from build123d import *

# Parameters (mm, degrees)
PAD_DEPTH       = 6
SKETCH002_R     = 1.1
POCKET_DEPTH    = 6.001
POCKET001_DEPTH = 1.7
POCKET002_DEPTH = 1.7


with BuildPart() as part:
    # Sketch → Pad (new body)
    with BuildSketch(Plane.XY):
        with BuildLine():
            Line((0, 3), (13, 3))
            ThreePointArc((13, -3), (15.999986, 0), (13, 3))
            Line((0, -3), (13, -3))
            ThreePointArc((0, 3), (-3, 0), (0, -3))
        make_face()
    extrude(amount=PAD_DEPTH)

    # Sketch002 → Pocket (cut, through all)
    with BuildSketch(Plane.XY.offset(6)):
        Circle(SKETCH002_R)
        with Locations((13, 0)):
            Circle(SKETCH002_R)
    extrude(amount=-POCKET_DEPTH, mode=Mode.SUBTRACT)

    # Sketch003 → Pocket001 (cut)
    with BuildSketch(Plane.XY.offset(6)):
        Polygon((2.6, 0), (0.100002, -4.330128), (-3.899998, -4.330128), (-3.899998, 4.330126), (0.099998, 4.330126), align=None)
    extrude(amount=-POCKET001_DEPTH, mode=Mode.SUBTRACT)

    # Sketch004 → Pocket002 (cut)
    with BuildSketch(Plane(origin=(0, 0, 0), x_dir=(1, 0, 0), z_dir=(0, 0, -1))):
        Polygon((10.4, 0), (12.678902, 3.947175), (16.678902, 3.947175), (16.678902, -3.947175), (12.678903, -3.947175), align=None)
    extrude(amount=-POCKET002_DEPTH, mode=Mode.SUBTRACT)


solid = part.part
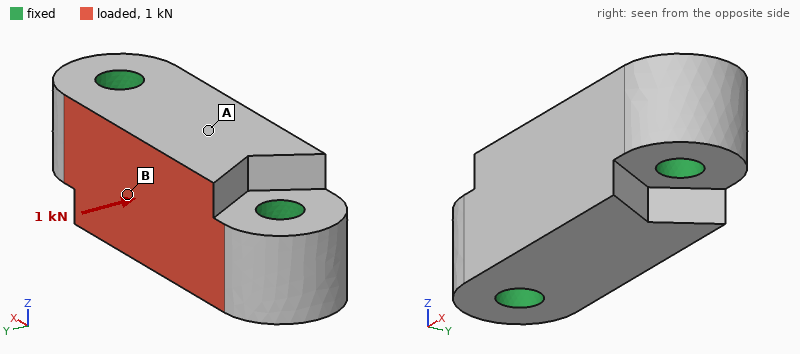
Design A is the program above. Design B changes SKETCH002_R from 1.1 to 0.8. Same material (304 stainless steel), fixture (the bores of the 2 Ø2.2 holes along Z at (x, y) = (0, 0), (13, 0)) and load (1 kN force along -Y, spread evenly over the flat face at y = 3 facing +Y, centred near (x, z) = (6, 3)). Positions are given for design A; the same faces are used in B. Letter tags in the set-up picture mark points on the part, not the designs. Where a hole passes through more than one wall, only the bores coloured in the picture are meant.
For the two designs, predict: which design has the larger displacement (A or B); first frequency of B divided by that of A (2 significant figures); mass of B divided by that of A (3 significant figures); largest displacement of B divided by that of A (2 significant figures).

B
0.88
1.03
1.2
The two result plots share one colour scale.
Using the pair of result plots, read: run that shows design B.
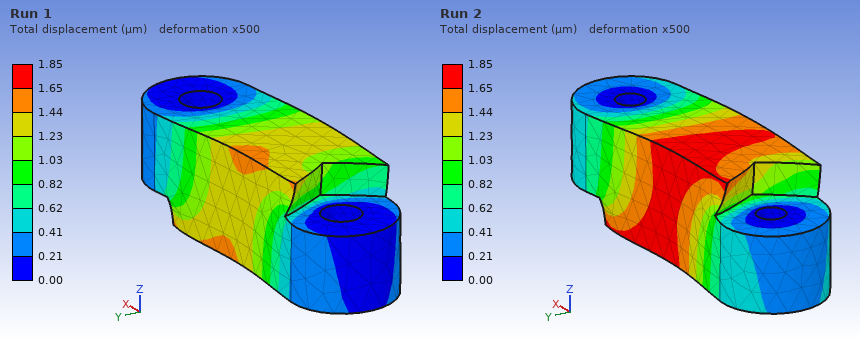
Run 2
